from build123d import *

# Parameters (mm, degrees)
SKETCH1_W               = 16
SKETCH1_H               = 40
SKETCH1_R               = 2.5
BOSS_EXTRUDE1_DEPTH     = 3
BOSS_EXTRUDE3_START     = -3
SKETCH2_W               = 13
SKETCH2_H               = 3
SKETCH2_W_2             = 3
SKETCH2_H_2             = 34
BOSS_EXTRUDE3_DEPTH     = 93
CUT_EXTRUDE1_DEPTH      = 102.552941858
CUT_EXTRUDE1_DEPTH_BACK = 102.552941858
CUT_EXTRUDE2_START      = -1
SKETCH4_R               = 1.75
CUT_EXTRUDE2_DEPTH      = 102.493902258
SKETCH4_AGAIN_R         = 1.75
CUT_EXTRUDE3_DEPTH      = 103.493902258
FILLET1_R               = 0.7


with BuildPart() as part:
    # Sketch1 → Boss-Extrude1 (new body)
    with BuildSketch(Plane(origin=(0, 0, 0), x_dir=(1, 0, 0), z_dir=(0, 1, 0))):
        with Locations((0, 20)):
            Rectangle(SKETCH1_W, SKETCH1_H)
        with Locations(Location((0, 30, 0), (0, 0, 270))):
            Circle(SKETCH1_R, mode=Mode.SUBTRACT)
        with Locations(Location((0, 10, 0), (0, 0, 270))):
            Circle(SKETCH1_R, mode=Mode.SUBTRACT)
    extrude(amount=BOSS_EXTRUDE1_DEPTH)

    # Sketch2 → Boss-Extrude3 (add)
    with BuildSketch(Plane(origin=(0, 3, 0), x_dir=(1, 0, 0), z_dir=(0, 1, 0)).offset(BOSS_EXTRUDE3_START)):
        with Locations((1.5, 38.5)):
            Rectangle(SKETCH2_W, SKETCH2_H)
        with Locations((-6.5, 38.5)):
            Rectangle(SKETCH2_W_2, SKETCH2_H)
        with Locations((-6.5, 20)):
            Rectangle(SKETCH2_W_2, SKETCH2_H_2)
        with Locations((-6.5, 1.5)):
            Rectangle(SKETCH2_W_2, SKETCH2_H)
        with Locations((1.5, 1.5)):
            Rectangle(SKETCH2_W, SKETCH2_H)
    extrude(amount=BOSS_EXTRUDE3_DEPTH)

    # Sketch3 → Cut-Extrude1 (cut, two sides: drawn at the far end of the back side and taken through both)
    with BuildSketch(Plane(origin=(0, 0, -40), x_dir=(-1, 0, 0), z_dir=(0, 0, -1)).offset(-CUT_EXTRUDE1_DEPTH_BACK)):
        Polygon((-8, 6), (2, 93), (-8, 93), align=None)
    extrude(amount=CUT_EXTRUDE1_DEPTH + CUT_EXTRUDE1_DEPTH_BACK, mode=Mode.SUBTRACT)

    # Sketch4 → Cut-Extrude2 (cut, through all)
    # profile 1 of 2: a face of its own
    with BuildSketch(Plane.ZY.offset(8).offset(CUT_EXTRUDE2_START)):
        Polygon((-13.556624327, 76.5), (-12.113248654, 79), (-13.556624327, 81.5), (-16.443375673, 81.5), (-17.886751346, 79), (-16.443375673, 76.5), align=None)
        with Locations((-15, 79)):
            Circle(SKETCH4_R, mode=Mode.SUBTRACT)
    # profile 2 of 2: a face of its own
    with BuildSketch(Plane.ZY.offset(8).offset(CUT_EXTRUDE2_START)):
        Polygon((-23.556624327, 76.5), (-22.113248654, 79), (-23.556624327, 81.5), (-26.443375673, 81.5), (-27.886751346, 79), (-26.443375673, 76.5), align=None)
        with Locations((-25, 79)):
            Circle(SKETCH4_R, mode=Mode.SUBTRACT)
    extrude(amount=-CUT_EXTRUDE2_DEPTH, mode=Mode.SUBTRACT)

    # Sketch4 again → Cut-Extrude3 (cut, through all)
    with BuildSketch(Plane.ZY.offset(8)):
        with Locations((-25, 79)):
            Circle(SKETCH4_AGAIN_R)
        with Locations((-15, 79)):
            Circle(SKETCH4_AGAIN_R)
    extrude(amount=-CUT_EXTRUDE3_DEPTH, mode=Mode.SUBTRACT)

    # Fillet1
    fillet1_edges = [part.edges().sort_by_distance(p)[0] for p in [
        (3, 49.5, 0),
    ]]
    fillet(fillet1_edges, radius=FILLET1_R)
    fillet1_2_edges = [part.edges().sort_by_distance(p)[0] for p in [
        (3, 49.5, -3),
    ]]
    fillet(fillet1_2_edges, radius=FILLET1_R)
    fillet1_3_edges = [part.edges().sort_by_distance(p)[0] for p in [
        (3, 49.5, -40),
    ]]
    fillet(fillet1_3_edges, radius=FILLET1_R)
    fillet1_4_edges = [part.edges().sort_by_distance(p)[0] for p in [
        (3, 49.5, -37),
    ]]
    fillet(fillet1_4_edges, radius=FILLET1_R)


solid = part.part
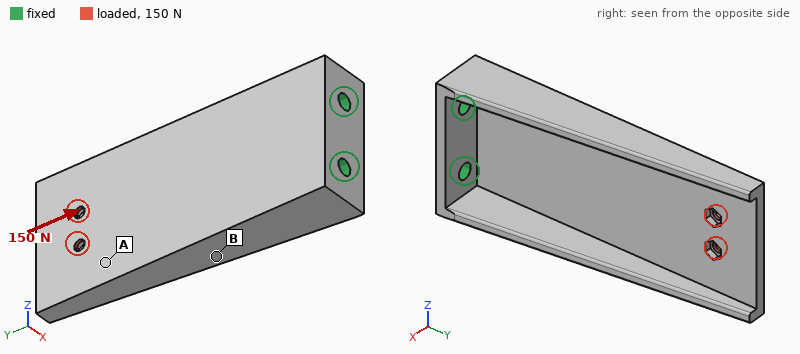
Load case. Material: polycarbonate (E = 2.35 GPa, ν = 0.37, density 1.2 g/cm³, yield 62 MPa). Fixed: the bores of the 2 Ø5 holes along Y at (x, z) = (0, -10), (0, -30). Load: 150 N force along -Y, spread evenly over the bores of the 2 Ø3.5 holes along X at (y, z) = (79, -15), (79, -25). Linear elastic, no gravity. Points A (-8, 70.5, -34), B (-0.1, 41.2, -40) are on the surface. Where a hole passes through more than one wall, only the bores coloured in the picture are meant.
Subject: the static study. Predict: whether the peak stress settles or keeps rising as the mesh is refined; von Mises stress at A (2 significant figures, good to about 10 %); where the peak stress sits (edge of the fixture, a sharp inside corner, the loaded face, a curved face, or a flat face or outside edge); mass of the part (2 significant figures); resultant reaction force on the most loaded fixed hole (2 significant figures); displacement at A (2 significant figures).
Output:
keeps rising
1.9 MPa
edge of the fixture
20 g
75 N
0.72 mm
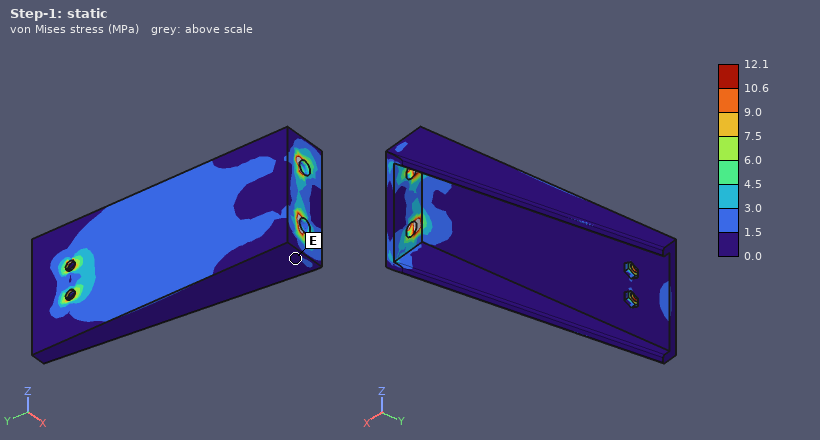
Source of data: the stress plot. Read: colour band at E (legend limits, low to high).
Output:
0.0 to 1.5 MPa
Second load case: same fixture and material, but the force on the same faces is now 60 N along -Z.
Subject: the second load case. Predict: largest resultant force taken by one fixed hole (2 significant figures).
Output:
190 N
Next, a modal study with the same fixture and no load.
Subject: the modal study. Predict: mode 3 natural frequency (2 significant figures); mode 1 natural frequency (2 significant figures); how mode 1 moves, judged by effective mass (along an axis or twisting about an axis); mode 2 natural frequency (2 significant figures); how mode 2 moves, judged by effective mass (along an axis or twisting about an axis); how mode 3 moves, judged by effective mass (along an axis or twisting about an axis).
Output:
690 Hz
200 Hz
along X
370 Hz
along Z
along Z
